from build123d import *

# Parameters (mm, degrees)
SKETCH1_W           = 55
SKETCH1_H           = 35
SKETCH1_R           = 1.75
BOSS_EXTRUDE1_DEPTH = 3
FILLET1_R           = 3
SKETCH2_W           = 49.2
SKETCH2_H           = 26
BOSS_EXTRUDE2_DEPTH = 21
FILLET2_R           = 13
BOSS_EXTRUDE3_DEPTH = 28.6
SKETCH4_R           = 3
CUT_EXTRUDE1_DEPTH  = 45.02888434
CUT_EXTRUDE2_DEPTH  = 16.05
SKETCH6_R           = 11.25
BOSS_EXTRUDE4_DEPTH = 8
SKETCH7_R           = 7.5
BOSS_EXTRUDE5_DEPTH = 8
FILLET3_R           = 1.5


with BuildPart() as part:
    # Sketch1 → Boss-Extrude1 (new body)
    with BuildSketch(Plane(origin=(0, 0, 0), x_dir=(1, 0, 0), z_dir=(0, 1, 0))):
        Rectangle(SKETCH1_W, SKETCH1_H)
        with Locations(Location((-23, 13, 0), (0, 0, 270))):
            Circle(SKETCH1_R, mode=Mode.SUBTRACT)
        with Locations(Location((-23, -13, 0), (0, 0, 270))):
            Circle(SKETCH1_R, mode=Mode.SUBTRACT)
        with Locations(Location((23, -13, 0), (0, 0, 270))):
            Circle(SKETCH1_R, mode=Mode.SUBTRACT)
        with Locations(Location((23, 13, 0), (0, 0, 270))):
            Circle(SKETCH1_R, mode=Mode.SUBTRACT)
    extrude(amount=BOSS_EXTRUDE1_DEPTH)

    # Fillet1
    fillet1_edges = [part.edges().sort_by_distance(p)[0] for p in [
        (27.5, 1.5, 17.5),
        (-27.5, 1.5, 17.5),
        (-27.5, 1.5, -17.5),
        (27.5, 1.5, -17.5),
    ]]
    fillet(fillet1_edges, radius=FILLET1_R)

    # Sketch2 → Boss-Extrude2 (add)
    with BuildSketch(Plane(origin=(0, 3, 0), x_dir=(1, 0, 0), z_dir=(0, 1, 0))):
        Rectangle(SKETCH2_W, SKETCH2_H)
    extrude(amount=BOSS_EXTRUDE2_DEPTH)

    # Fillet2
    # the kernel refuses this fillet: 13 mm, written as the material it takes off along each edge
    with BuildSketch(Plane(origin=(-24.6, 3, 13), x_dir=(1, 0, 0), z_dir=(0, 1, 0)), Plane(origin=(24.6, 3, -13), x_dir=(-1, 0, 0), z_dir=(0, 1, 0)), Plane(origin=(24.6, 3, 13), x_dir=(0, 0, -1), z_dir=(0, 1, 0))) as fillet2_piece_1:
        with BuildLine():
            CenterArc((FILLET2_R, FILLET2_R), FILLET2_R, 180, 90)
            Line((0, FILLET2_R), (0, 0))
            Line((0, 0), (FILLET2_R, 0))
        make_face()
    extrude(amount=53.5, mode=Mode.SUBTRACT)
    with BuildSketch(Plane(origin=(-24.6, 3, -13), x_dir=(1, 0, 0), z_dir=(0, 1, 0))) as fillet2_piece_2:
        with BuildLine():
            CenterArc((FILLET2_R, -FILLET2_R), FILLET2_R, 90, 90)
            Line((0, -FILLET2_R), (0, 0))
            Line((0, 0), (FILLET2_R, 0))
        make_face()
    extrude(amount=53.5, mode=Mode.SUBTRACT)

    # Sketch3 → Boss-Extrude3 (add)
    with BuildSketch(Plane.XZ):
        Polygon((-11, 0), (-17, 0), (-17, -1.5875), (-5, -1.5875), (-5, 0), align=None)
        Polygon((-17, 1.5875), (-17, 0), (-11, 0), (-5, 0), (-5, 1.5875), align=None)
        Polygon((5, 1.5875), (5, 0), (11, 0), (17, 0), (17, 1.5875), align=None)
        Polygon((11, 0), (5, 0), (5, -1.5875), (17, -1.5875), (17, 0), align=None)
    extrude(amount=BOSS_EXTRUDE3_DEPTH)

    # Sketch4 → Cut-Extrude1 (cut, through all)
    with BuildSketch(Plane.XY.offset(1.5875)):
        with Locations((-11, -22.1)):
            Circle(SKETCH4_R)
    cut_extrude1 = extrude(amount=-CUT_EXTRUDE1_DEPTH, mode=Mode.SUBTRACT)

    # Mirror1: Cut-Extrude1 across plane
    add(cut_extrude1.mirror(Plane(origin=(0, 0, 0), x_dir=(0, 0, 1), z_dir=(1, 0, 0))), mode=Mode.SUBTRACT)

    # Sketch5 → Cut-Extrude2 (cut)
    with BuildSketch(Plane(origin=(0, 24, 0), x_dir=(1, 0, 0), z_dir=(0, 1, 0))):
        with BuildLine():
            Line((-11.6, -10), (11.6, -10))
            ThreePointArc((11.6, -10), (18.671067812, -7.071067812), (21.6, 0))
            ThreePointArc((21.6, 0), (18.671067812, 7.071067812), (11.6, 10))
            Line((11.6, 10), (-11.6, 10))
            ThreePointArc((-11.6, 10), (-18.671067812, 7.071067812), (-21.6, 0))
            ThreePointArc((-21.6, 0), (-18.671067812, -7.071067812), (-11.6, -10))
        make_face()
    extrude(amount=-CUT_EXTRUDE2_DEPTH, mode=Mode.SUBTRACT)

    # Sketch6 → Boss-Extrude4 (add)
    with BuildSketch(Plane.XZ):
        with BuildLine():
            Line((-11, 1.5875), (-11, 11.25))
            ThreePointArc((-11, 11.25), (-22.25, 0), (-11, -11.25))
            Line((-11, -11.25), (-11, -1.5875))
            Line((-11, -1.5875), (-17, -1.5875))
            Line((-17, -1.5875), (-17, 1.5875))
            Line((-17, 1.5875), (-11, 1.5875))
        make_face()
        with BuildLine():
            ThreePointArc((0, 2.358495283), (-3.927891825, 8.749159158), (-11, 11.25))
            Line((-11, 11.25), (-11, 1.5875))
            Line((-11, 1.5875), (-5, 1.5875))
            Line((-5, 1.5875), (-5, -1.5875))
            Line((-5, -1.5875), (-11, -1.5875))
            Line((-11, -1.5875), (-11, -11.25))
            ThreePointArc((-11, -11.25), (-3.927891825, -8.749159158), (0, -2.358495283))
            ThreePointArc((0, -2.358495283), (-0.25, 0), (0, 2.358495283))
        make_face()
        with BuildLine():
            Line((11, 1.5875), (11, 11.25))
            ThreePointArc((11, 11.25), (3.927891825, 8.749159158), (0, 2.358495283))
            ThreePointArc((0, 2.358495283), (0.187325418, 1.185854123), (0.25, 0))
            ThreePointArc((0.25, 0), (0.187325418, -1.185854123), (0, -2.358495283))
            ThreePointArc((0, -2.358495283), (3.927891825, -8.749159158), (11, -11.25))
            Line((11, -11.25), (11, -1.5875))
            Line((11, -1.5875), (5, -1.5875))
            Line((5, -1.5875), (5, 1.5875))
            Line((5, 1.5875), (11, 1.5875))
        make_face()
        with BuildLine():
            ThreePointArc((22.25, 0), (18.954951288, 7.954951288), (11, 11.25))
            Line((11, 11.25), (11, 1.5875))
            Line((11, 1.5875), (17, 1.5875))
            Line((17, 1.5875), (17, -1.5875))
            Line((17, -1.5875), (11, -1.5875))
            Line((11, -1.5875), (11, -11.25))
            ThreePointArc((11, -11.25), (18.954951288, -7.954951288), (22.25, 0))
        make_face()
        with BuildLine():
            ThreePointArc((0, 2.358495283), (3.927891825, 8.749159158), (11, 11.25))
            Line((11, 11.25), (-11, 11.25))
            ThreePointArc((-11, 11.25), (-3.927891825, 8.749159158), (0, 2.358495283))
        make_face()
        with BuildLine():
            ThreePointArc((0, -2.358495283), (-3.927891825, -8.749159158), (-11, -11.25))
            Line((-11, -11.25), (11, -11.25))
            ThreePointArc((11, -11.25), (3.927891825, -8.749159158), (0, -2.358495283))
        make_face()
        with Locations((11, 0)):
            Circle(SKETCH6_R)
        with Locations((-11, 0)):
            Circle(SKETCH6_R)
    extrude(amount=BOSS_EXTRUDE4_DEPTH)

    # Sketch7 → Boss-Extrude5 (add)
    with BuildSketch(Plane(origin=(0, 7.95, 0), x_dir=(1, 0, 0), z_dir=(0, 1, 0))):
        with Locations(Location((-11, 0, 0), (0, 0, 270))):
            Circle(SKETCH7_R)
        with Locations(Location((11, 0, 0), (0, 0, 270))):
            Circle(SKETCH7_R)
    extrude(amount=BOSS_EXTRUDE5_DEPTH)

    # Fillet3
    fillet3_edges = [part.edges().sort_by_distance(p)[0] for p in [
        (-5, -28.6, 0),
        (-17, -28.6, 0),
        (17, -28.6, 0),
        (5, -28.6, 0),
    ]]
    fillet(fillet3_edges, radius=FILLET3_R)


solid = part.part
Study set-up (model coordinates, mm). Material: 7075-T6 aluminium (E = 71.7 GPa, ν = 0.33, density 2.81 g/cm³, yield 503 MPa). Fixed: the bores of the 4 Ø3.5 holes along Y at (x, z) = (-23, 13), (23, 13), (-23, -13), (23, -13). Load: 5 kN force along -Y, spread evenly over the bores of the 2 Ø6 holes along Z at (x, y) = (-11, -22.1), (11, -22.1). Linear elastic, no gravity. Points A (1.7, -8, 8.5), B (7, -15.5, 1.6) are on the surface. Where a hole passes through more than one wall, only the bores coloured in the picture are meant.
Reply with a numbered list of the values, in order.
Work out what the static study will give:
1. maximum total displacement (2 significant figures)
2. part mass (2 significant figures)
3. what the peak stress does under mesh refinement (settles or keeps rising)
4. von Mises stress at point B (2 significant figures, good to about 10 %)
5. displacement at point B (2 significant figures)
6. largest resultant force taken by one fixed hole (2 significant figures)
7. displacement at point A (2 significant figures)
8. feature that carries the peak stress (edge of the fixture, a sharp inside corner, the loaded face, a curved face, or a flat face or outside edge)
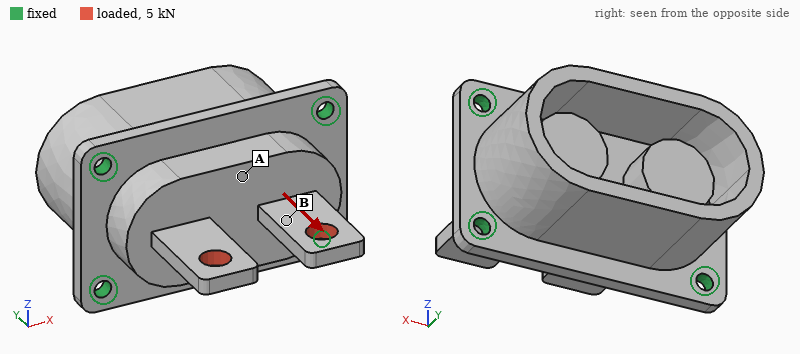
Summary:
1. 46 µm
2. 80 g
3. keeps rising
4. 70 MPa
5. 30 µm
6. 1.3 kN
7. 21 µm
8. edge of the fixture
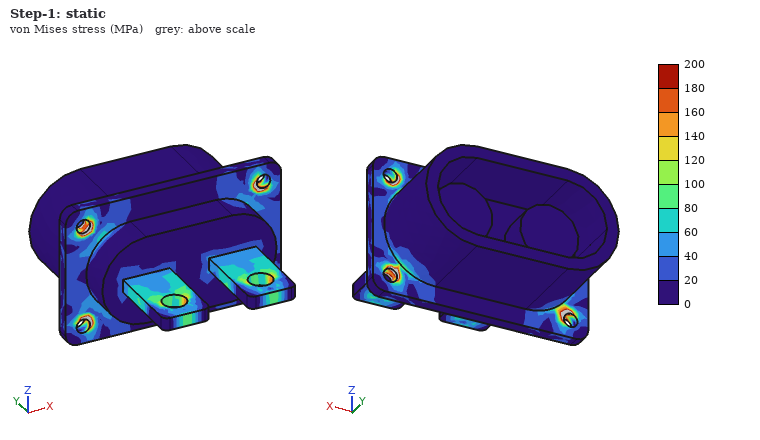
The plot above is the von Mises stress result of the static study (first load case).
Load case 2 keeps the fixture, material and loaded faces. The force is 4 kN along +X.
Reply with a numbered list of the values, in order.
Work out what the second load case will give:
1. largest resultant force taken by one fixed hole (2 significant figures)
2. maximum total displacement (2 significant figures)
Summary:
1. 1.5 kN
2. 0.23 mm
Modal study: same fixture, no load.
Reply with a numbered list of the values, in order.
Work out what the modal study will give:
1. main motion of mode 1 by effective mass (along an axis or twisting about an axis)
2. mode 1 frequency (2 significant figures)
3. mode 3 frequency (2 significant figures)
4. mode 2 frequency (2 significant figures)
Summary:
1. twisting about X
2. 5800 Hz
3. 9100 Hz
4. 6100 Hz
